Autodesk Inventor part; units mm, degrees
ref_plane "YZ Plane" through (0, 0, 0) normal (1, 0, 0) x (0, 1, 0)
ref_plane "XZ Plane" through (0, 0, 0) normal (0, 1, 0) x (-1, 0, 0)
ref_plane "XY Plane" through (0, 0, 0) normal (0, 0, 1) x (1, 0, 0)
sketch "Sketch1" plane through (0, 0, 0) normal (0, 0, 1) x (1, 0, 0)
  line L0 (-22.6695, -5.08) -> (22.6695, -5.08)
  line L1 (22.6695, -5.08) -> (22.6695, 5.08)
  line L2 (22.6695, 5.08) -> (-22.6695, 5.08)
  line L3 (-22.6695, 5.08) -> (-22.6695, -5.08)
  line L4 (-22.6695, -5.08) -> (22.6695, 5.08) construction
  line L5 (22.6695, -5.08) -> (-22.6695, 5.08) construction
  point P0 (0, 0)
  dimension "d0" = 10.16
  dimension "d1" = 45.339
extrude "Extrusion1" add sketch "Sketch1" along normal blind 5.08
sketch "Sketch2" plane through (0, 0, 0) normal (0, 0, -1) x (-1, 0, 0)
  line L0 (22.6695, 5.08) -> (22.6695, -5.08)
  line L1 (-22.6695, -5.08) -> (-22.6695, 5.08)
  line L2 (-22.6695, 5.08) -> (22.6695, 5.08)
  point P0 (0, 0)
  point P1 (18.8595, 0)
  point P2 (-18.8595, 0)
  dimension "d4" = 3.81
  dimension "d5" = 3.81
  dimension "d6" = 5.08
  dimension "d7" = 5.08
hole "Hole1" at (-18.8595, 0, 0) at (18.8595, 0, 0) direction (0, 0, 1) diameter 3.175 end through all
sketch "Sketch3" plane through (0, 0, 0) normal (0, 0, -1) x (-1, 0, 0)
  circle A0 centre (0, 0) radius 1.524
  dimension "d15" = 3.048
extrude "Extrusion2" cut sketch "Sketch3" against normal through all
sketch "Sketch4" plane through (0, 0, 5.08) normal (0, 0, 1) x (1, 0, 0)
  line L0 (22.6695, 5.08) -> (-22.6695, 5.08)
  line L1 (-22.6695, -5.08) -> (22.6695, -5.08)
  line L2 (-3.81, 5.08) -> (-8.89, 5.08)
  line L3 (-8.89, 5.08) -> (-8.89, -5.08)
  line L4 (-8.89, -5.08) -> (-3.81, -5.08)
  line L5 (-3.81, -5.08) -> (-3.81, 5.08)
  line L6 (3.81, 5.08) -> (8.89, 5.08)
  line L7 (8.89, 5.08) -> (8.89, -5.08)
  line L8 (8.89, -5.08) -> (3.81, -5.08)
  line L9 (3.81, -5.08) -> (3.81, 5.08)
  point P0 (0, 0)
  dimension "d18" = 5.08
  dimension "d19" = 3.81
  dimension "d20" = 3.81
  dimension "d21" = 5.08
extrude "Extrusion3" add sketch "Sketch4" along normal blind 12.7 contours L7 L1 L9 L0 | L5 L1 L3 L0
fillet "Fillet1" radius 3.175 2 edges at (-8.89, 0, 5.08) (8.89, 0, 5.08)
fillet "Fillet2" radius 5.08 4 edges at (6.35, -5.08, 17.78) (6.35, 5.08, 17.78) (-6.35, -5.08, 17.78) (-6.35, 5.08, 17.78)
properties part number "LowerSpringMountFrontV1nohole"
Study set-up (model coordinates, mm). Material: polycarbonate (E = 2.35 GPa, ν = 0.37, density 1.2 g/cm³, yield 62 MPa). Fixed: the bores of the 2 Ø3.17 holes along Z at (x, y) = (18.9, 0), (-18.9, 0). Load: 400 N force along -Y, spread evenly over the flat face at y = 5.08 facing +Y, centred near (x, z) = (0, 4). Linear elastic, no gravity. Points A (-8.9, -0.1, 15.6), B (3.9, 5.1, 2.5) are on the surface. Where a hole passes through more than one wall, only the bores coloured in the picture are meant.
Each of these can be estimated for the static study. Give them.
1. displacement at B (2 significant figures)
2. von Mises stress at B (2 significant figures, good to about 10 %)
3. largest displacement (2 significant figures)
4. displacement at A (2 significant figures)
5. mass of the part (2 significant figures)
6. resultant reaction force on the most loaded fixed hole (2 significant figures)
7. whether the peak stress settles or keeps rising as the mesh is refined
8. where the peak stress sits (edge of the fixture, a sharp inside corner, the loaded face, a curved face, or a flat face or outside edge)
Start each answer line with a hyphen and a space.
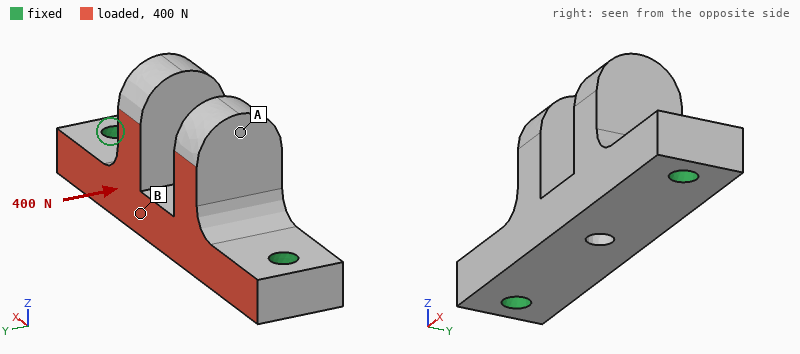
- 0.13 mm
- 8.8 MPa
- 0.30 mm
- 0.25 mm
- 4.2 g
- 200 N
- keeps rising
- edge of the fixture
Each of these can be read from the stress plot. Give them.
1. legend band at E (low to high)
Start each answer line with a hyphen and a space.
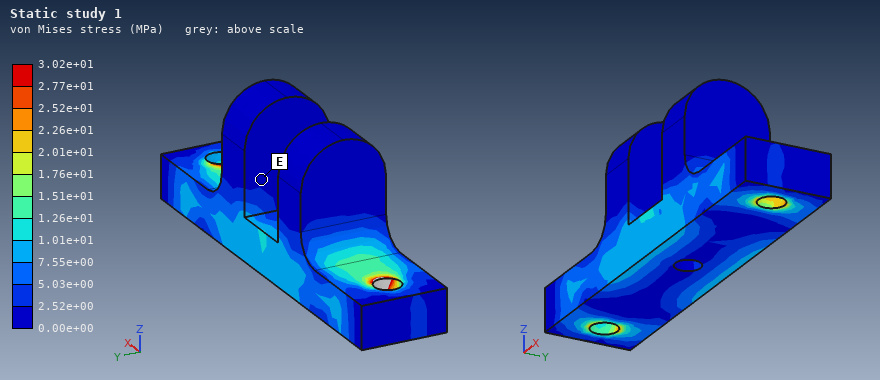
- 0.00e+00 to 2.52e+00 MPa
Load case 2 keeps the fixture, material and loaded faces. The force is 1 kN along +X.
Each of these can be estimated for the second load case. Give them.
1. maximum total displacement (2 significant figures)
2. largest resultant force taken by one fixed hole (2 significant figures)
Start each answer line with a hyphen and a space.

- 0.15 mm
- 520 N
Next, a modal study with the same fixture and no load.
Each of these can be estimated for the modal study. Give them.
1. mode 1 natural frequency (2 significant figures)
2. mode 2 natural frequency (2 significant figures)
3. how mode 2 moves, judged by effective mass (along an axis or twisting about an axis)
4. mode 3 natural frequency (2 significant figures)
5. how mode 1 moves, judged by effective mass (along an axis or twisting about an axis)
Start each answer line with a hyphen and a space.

- 2800 Hz
- 3000 Hz
- along Z
- 4700 Hz
- along Y
